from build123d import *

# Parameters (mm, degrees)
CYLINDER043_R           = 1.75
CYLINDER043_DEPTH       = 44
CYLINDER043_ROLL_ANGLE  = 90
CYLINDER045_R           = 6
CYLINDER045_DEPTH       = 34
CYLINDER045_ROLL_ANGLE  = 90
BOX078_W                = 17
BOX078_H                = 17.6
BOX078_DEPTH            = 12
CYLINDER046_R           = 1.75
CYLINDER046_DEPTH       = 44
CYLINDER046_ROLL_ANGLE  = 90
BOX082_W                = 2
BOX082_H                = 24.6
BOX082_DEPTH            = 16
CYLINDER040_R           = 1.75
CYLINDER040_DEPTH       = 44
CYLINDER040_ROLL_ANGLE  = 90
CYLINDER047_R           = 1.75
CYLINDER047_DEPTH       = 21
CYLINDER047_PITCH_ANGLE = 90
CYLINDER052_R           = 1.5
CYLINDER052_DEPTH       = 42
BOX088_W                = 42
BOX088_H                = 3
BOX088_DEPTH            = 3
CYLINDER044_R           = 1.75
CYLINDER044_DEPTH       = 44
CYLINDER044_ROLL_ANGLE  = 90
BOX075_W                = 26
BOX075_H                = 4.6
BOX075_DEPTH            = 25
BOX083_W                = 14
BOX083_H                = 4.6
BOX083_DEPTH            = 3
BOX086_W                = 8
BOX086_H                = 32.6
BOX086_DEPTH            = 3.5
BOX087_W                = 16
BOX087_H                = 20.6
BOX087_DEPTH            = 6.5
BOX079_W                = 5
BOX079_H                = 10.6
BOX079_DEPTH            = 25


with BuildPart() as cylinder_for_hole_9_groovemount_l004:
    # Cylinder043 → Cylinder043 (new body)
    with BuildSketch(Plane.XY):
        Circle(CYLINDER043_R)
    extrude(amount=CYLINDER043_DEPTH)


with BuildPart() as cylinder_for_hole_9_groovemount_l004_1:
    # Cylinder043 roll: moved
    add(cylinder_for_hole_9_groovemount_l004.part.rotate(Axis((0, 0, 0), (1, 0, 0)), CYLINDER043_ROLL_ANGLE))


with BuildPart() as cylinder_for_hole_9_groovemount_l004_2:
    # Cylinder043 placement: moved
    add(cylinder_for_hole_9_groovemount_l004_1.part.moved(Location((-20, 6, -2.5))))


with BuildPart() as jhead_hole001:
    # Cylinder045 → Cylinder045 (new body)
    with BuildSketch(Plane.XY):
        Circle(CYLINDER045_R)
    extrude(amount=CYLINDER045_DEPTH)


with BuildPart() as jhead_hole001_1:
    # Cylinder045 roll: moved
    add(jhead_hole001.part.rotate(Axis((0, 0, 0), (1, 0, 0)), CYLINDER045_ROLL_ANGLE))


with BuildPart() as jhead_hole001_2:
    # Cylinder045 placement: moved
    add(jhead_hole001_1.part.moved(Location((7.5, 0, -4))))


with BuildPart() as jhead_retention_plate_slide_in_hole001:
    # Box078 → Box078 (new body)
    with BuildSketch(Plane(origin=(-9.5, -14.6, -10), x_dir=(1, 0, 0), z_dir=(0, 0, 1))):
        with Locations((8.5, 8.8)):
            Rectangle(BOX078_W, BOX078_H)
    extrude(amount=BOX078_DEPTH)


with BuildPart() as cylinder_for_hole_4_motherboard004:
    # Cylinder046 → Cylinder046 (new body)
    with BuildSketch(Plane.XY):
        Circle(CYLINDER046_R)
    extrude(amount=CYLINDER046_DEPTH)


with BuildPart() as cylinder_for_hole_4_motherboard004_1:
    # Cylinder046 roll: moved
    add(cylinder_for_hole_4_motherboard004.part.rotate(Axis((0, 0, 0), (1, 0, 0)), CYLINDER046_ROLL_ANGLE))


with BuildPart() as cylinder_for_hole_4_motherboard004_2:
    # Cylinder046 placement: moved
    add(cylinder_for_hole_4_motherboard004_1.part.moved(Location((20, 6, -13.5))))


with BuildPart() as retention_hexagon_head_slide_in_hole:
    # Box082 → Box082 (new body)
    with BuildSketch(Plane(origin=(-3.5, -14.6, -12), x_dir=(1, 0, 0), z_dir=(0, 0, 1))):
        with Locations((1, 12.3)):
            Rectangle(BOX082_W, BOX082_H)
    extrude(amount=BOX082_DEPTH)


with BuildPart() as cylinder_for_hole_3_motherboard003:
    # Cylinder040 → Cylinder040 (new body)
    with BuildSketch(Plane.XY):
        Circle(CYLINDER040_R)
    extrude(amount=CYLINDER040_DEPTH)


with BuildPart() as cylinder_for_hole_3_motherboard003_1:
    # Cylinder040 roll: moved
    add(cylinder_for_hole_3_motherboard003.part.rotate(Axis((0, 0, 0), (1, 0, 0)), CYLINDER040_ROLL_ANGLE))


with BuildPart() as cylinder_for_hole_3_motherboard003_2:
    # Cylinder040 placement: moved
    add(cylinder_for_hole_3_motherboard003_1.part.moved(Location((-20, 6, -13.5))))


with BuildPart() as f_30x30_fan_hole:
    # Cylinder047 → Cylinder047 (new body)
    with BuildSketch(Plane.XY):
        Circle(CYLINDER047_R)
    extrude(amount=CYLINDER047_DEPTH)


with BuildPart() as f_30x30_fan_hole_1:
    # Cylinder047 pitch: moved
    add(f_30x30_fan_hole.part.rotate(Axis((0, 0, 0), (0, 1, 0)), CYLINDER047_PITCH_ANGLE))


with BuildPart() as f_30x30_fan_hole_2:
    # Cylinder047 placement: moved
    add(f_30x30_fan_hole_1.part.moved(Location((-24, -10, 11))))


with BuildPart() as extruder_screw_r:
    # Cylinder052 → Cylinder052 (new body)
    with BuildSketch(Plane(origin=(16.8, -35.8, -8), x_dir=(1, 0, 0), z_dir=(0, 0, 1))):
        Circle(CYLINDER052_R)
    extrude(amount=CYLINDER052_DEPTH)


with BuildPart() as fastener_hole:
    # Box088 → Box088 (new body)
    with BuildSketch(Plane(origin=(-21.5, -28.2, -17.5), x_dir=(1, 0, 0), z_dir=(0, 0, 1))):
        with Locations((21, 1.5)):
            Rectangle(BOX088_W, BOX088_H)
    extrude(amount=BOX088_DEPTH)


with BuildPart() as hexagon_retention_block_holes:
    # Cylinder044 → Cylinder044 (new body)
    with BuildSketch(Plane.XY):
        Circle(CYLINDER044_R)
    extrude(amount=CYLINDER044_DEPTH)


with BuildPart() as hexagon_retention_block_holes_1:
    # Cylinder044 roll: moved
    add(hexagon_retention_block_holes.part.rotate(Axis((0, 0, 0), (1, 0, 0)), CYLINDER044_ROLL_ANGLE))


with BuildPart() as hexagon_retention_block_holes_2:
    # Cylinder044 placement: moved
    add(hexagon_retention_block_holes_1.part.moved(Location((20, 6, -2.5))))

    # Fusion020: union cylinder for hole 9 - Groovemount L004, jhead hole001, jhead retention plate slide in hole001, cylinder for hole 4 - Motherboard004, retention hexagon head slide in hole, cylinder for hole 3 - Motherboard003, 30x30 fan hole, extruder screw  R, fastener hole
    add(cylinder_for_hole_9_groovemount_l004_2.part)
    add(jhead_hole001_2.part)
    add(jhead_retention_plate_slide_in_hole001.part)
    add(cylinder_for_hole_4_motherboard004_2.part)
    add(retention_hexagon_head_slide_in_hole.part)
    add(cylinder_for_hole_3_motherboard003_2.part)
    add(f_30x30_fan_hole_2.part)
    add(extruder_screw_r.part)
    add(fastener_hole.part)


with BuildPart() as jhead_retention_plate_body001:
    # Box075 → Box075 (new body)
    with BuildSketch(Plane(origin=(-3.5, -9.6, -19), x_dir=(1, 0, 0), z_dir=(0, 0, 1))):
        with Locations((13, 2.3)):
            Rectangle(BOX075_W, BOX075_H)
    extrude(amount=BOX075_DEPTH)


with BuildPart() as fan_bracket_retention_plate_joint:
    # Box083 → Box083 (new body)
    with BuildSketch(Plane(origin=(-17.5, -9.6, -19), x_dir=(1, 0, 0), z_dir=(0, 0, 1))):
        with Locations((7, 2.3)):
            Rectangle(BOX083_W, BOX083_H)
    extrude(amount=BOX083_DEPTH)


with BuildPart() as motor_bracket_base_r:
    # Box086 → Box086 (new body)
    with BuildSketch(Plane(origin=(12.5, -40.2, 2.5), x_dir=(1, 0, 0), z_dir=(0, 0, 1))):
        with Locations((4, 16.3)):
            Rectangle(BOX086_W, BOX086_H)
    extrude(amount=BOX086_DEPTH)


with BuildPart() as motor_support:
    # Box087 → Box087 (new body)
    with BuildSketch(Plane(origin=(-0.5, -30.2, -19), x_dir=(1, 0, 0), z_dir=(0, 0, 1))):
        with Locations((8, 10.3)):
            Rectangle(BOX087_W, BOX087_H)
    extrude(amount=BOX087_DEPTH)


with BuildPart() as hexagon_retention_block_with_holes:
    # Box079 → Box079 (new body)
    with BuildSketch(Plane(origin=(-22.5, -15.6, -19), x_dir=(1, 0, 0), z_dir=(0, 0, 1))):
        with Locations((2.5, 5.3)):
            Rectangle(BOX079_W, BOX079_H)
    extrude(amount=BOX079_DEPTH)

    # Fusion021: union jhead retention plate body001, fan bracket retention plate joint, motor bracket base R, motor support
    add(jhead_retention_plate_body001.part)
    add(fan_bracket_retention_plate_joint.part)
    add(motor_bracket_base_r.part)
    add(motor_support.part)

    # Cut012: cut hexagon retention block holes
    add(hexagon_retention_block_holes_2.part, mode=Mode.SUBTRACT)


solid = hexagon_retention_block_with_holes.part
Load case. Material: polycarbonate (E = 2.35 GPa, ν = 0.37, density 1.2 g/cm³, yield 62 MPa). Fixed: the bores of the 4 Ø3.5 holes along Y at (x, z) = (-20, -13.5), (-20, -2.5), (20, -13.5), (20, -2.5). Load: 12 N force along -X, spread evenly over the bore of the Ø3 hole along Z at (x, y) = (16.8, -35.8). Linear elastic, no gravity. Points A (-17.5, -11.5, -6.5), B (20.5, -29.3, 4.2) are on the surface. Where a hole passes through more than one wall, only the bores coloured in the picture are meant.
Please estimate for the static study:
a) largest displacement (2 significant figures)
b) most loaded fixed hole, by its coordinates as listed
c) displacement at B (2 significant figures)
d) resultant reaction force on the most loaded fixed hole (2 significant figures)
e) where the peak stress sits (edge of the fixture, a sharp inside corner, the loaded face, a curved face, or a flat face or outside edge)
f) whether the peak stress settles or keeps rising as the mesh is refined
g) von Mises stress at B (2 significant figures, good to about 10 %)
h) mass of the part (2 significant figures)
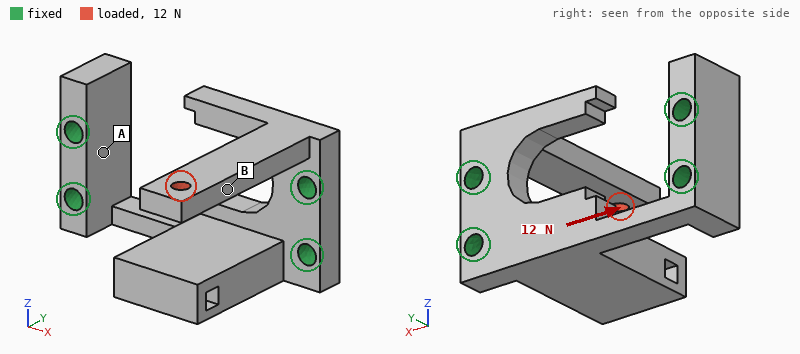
0.63 mm
(20, -2.5)
0.38 mm
16 N
edge of the fixture
keeps rising
2.1 MPa
7.4 g
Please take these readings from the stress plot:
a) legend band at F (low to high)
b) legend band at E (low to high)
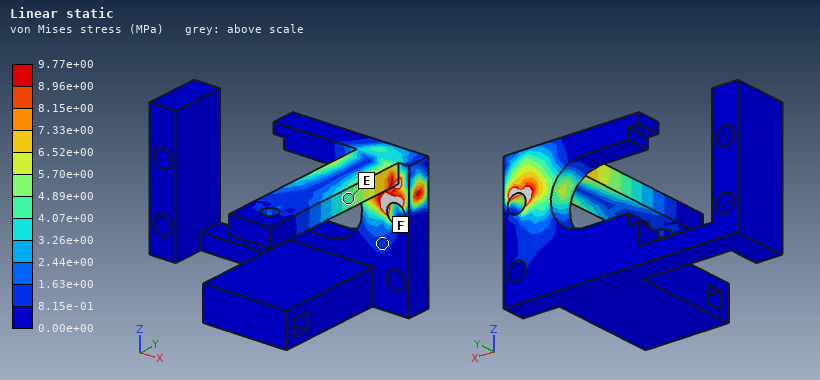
8.15e-01 to 1.63e+00 MPa
4.07e+00 to 4.89e+00 MPa
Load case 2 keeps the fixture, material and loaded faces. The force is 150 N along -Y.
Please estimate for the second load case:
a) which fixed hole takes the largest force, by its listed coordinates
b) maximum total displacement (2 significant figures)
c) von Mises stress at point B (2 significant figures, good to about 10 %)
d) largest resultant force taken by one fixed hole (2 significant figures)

(20, -2.5)
0.67 mm
6.8 MPa
160 N
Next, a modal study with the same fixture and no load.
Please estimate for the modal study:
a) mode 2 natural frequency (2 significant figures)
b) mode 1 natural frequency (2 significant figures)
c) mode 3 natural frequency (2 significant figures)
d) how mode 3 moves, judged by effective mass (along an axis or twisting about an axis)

1100 Hz
720 Hz
1400 Hz
along Z
